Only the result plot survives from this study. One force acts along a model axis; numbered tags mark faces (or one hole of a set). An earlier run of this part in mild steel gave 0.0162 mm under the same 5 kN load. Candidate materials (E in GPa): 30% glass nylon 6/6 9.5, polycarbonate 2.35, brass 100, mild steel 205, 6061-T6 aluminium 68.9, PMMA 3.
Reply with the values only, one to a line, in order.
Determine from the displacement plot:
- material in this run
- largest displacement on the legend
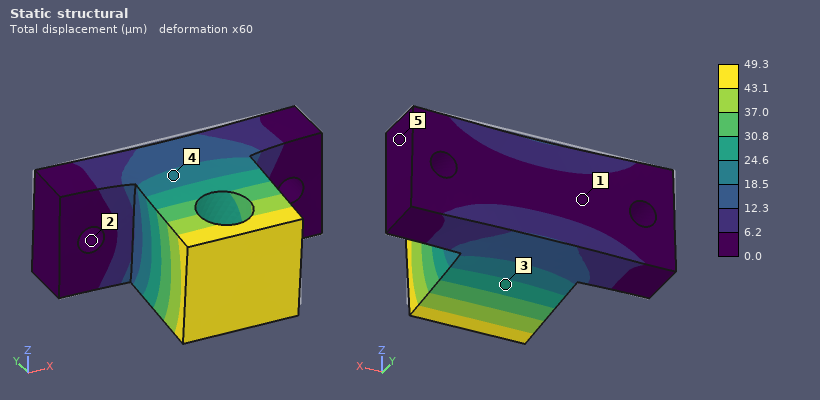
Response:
6061-T6 aluminium
49.3 µm
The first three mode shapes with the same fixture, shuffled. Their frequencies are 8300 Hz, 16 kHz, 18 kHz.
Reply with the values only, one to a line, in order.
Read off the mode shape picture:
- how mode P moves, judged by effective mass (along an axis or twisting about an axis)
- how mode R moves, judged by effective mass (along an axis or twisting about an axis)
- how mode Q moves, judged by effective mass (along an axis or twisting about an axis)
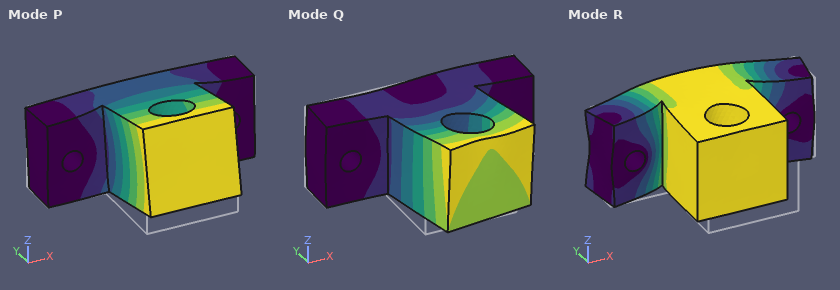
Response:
along Z
along Y
along X
